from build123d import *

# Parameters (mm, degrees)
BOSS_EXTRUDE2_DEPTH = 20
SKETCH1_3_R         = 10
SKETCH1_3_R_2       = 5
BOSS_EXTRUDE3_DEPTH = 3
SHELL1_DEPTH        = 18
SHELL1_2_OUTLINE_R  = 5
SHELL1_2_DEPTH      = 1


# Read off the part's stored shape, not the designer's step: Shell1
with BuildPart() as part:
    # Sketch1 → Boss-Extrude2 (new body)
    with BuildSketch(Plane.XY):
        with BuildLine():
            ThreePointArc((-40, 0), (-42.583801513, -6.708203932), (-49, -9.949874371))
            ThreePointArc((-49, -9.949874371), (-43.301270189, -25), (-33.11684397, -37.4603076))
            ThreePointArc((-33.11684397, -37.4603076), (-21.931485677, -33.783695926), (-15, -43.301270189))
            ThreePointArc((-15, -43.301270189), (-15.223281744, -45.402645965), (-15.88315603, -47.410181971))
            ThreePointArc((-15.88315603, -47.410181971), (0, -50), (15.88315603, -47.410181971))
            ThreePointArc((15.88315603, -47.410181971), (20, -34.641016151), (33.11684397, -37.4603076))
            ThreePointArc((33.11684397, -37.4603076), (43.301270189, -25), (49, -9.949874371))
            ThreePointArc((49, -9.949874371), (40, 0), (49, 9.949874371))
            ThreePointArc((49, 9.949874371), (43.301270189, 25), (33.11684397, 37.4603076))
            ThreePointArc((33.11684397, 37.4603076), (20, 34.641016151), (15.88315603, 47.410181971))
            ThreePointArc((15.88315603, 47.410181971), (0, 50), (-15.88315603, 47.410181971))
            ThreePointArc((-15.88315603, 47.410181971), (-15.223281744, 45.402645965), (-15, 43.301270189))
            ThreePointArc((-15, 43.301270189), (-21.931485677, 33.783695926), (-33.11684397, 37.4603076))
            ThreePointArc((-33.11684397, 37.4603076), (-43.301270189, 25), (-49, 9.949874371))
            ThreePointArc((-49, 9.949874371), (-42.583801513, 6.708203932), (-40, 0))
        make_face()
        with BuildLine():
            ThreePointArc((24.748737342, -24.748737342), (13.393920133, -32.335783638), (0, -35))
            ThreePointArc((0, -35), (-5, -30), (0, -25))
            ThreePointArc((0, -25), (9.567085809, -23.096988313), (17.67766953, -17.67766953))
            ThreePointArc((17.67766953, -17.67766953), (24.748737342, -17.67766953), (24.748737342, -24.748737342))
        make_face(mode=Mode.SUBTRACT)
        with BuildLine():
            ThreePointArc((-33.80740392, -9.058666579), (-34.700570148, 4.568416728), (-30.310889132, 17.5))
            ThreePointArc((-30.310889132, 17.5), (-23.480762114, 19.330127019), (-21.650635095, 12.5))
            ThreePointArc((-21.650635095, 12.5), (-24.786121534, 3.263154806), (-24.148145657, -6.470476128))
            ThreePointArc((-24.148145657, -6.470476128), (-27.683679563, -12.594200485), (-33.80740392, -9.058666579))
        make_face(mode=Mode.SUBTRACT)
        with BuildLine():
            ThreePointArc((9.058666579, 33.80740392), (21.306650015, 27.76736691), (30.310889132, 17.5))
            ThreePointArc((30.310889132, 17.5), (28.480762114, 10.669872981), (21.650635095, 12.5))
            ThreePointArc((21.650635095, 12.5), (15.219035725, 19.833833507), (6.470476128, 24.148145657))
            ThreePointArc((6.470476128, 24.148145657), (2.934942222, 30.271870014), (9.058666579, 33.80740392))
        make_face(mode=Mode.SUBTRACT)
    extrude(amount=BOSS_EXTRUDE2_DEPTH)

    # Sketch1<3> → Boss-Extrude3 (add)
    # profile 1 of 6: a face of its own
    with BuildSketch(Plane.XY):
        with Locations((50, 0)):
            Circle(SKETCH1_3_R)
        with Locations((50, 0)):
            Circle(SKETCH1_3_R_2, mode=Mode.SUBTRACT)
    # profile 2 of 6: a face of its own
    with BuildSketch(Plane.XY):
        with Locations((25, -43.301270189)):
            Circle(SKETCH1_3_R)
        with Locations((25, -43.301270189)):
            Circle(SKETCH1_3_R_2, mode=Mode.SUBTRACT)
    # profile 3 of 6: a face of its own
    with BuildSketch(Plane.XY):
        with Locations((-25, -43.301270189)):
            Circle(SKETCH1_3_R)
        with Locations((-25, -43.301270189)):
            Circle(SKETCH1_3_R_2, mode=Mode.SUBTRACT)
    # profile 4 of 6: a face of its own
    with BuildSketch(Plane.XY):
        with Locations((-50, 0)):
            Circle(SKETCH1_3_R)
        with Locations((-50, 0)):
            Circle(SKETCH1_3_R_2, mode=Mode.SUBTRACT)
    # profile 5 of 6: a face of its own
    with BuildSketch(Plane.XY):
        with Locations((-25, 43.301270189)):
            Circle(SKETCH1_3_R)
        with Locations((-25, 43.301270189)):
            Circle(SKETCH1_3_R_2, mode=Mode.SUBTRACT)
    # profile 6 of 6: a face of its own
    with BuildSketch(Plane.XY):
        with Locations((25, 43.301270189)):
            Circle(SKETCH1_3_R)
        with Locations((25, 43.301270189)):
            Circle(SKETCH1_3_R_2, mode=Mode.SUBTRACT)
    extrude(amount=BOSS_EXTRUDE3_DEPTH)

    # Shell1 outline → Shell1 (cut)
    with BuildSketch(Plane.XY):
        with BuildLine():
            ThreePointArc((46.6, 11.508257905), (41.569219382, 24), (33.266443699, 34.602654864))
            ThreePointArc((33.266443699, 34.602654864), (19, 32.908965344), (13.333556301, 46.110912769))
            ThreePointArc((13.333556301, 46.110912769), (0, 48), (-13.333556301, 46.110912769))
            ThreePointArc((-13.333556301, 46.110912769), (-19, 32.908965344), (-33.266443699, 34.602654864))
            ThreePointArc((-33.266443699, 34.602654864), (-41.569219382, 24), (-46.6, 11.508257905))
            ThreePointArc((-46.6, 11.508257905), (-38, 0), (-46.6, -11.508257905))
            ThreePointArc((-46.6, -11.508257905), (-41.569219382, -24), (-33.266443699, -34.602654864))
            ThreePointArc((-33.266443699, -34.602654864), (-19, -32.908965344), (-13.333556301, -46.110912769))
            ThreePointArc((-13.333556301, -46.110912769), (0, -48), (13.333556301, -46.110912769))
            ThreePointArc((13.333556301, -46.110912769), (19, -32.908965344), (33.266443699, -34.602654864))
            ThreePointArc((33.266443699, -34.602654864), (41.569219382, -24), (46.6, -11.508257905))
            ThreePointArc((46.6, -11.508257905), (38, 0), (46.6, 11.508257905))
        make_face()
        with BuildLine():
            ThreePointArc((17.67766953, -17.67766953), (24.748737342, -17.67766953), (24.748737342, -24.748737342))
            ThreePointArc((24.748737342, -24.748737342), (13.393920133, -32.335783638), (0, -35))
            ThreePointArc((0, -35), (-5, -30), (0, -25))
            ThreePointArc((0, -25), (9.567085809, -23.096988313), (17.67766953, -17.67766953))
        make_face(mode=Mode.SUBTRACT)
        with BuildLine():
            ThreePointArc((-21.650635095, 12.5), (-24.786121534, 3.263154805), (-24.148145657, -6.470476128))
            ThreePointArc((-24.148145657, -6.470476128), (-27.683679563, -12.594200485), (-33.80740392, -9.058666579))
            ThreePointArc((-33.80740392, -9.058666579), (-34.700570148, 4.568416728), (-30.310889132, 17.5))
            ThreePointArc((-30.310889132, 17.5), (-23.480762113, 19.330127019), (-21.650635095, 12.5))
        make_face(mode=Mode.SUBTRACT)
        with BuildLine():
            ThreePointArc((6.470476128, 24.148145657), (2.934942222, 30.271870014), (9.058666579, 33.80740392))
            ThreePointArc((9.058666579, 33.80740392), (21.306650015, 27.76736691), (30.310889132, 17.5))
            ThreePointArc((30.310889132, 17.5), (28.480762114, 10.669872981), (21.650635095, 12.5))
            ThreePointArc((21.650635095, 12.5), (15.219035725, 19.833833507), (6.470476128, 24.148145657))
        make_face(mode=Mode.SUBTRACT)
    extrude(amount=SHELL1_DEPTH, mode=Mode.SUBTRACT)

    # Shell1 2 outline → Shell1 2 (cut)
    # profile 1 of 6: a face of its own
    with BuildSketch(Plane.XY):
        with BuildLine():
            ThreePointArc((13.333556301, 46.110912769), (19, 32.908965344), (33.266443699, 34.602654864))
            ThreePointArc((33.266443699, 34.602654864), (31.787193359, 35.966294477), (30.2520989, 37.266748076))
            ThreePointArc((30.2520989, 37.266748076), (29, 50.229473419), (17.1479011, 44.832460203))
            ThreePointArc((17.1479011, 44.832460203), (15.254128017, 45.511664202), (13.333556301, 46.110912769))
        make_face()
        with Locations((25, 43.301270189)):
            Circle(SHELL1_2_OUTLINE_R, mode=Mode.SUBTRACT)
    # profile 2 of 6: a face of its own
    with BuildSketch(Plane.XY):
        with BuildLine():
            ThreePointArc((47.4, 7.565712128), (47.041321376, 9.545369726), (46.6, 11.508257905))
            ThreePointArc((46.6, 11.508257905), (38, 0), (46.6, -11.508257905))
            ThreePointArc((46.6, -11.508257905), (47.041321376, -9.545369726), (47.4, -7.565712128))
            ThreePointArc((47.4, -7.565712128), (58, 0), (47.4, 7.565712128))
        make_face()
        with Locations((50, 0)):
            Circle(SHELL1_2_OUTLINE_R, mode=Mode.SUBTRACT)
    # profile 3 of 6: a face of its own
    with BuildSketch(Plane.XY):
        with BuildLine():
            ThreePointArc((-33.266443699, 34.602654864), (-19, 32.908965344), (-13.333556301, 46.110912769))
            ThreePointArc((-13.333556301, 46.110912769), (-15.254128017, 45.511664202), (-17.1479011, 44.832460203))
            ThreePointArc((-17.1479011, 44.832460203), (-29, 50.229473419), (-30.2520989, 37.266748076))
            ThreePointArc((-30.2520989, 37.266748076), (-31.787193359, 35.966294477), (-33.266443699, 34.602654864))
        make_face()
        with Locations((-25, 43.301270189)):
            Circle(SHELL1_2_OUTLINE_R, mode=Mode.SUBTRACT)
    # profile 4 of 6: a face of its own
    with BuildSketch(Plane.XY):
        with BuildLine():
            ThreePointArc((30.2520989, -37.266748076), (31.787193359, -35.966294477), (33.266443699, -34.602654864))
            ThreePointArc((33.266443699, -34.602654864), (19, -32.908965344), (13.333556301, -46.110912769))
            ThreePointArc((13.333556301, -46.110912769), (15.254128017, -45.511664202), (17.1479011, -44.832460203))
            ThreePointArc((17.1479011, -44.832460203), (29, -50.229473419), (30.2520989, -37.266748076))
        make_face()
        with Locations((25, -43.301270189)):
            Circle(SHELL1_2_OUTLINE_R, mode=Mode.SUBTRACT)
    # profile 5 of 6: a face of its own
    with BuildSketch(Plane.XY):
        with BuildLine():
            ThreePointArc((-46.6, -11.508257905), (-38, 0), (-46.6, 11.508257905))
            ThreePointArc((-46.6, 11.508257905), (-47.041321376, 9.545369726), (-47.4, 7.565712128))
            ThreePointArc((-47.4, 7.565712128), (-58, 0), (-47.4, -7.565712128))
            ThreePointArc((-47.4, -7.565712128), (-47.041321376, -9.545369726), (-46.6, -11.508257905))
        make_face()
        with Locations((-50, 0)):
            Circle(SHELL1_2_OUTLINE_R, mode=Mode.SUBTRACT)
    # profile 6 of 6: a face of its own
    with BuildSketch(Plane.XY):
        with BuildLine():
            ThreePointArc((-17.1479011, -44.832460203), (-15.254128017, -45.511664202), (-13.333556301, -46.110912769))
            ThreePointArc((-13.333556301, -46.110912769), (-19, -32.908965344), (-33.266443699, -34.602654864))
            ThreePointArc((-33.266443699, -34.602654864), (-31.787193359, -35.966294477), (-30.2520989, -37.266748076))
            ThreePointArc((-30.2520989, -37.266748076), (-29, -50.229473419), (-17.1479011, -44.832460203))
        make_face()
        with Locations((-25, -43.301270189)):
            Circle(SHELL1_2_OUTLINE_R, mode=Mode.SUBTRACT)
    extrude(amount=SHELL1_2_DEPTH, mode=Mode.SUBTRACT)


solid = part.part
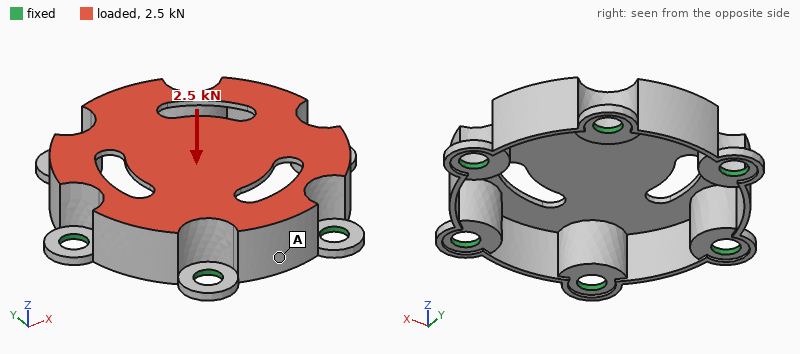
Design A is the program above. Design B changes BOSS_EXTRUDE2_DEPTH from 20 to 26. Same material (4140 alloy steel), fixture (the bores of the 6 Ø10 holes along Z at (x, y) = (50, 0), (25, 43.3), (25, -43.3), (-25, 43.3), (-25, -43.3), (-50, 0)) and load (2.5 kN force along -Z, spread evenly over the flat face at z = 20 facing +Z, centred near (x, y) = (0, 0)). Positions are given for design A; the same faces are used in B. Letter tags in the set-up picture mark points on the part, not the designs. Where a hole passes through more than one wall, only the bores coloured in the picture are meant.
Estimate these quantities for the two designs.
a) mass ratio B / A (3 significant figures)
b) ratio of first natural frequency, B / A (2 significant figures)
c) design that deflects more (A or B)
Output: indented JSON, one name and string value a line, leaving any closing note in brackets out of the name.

{
  "mass ratio B / A": "2.30",
  "ratio of first natural frequency, B / A": "2.2",
  "design that deflects more": "A"
}
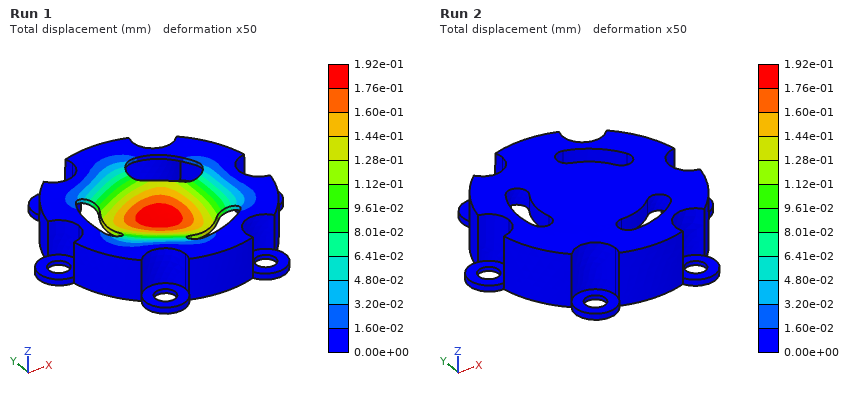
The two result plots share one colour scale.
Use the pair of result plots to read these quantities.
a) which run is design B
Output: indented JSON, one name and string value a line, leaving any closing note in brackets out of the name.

{
  "which run is design B": "Run 2"
}
